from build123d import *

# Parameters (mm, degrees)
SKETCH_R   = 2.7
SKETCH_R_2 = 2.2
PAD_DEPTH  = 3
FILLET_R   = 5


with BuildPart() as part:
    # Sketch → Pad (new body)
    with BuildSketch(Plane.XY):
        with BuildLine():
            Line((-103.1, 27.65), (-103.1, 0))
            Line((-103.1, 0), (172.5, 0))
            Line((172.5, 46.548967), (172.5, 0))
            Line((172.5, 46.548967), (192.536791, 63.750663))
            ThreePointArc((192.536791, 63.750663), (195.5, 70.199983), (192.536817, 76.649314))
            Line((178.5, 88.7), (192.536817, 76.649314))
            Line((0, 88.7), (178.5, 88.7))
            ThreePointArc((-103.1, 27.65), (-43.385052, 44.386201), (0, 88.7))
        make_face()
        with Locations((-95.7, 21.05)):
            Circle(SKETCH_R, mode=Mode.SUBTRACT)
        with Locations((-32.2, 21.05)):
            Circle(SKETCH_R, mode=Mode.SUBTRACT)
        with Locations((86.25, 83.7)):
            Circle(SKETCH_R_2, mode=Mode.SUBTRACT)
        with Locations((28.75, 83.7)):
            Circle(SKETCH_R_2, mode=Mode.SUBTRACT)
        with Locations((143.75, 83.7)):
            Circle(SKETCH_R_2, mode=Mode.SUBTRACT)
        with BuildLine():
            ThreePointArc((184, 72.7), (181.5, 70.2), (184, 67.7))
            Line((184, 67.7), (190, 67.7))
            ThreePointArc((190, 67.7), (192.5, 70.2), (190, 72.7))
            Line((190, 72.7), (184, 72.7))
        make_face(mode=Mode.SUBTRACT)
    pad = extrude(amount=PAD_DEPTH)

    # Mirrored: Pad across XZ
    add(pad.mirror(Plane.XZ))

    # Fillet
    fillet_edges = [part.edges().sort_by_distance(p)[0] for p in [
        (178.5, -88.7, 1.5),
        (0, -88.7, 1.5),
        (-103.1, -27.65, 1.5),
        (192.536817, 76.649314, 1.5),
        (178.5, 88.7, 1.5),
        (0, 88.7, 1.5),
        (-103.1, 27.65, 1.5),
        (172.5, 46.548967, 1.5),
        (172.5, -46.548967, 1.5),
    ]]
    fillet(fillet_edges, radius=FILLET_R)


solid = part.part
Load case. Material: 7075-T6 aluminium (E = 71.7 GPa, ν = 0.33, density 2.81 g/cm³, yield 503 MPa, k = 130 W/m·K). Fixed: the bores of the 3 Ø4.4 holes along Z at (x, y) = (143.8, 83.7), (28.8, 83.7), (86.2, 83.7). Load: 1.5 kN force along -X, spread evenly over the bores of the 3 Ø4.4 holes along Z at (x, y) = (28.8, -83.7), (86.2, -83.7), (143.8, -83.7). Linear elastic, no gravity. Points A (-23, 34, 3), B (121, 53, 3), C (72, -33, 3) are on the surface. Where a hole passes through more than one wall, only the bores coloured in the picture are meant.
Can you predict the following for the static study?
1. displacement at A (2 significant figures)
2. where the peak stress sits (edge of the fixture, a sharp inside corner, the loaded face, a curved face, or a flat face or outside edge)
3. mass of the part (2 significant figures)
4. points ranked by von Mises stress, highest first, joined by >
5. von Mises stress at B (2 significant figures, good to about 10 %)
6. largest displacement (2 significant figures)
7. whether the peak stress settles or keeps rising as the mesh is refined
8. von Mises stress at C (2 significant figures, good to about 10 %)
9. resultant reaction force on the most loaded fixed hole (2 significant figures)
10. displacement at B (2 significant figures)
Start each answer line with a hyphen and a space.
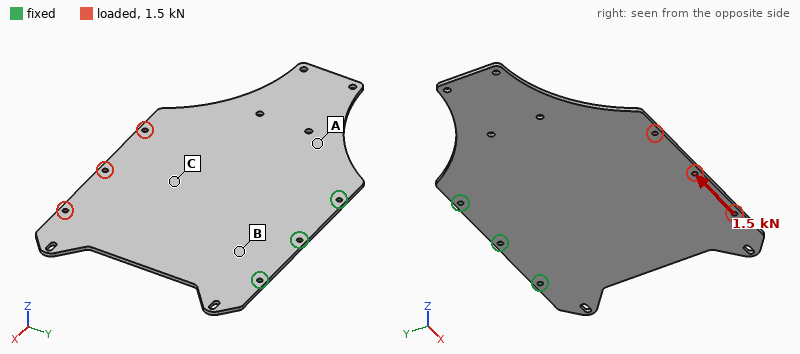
- 44 µm
- edge of the fixture
- 350 g
- B > C > A
- 12 MPa
- 87 µm
- keeps rising
- 7.0 MPa
- 2.2 kN
- 14 µm
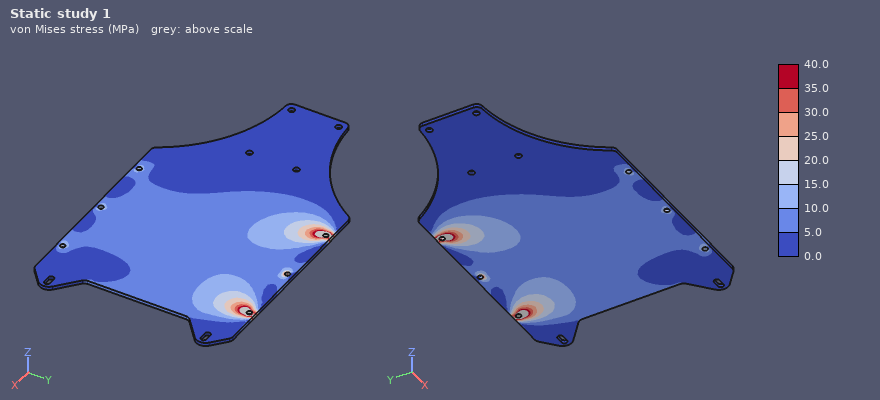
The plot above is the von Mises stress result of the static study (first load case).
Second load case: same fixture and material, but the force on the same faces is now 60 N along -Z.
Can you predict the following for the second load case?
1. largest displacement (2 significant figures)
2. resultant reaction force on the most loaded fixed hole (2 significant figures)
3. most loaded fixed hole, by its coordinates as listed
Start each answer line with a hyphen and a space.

- 3.5 mm
- 38 N
- (86.2, 83.7)
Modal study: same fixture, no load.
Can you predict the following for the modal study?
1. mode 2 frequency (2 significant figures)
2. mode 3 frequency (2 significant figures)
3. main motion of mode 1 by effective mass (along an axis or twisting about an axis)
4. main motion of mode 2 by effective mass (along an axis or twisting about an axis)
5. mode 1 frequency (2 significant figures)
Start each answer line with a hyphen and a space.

- 110 Hz
- 250 Hz
- along Z
- twisting about Y
- 71 Hz
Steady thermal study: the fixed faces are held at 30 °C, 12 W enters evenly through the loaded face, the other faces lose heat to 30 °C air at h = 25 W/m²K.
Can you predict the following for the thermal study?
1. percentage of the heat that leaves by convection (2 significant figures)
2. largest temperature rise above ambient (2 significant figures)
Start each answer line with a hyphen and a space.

- 80 %
- 17 K
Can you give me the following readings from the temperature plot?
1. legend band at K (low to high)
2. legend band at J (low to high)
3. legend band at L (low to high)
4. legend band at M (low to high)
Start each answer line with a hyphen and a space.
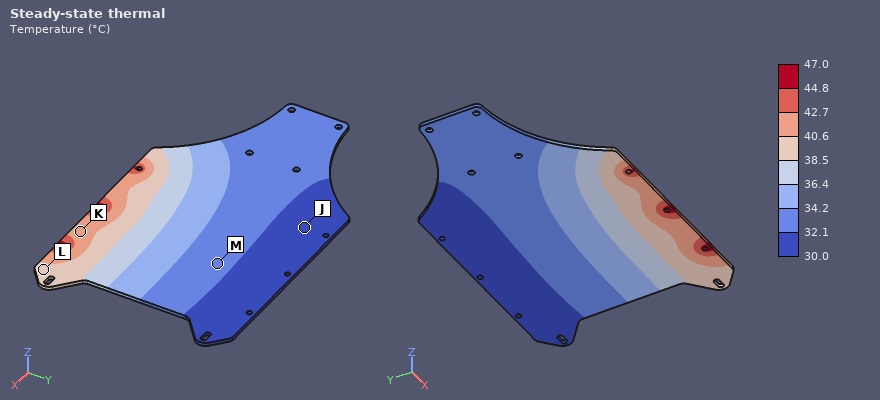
- 40.6 to 42.7 °C
- 30.0 to 32.1 °C
- 38.5 to 40.6 °C
- 32.1 to 34.2 °C
